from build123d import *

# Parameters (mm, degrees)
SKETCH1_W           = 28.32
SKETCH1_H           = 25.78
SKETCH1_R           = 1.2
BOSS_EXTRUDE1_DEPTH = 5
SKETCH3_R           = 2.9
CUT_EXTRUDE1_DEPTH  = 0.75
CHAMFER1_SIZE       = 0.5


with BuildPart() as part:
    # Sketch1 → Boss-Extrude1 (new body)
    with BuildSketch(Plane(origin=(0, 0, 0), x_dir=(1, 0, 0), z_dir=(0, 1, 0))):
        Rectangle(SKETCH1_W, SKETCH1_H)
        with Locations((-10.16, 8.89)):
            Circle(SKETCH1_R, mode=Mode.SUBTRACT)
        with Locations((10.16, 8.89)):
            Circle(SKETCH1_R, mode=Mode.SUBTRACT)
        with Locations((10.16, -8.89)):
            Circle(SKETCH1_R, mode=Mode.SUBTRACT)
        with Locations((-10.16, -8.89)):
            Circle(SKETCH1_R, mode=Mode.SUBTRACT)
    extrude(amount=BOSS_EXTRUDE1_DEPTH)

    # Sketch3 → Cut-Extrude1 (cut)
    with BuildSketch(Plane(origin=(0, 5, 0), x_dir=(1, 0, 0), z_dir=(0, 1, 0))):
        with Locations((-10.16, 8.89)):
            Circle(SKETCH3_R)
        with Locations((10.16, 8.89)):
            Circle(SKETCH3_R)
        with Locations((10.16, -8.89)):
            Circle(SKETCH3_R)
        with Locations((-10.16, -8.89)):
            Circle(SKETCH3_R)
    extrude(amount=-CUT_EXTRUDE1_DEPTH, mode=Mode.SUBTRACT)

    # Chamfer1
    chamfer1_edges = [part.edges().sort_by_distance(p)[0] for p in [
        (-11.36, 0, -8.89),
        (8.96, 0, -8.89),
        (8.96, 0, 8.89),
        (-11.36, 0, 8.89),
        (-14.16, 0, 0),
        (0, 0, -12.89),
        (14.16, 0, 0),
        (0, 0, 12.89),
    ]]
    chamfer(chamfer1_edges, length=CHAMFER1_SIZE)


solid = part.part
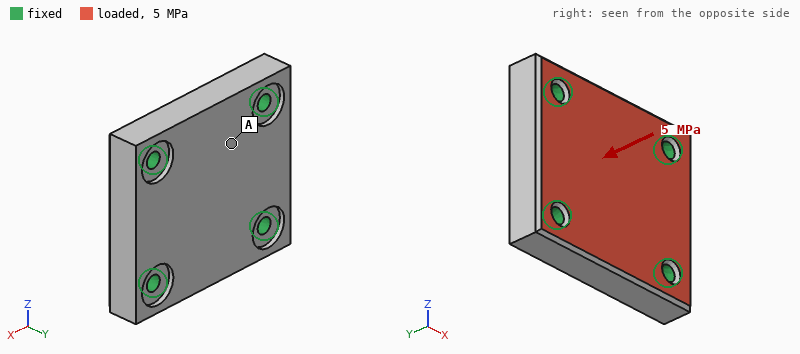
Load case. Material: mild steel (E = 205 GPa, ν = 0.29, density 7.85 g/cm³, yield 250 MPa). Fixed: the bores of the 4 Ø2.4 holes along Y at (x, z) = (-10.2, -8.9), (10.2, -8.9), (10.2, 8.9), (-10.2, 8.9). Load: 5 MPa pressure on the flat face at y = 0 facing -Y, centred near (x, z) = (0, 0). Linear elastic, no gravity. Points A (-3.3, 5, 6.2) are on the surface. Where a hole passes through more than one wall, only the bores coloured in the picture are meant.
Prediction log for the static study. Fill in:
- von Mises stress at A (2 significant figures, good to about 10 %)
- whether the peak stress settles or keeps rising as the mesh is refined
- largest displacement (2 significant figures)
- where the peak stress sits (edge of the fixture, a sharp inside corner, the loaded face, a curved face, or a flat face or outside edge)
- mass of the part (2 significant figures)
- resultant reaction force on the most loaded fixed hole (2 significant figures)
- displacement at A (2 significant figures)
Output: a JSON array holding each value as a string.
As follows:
["21 MPa", "keeps rising", "3.5 µm", "edge of the fixture", "27 g", "800 N", "2.7 µm"]
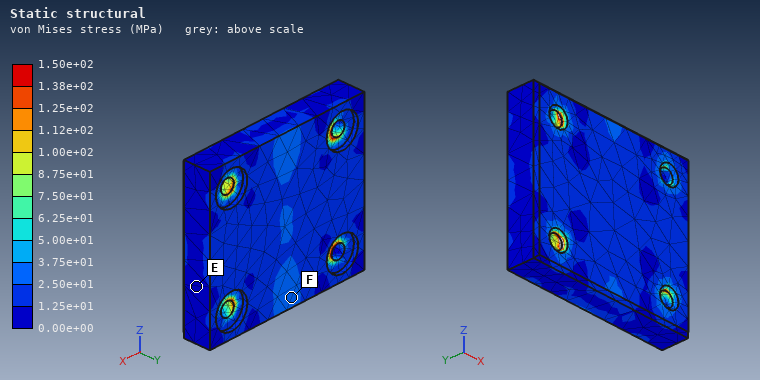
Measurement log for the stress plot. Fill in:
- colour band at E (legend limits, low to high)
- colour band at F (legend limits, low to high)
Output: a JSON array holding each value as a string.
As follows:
["0.00e+00 to 1.25e+01 MPa", "2.50e+01 to 3.75e+01 MPa"]
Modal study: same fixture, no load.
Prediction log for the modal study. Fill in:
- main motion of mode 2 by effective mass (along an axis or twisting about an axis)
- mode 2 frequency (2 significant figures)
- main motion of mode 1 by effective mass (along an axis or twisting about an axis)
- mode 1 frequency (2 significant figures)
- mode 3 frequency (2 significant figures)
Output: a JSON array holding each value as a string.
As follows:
["twisting about X", "47 kHz", "along Y", "35 kHz", "53 kHz"]
